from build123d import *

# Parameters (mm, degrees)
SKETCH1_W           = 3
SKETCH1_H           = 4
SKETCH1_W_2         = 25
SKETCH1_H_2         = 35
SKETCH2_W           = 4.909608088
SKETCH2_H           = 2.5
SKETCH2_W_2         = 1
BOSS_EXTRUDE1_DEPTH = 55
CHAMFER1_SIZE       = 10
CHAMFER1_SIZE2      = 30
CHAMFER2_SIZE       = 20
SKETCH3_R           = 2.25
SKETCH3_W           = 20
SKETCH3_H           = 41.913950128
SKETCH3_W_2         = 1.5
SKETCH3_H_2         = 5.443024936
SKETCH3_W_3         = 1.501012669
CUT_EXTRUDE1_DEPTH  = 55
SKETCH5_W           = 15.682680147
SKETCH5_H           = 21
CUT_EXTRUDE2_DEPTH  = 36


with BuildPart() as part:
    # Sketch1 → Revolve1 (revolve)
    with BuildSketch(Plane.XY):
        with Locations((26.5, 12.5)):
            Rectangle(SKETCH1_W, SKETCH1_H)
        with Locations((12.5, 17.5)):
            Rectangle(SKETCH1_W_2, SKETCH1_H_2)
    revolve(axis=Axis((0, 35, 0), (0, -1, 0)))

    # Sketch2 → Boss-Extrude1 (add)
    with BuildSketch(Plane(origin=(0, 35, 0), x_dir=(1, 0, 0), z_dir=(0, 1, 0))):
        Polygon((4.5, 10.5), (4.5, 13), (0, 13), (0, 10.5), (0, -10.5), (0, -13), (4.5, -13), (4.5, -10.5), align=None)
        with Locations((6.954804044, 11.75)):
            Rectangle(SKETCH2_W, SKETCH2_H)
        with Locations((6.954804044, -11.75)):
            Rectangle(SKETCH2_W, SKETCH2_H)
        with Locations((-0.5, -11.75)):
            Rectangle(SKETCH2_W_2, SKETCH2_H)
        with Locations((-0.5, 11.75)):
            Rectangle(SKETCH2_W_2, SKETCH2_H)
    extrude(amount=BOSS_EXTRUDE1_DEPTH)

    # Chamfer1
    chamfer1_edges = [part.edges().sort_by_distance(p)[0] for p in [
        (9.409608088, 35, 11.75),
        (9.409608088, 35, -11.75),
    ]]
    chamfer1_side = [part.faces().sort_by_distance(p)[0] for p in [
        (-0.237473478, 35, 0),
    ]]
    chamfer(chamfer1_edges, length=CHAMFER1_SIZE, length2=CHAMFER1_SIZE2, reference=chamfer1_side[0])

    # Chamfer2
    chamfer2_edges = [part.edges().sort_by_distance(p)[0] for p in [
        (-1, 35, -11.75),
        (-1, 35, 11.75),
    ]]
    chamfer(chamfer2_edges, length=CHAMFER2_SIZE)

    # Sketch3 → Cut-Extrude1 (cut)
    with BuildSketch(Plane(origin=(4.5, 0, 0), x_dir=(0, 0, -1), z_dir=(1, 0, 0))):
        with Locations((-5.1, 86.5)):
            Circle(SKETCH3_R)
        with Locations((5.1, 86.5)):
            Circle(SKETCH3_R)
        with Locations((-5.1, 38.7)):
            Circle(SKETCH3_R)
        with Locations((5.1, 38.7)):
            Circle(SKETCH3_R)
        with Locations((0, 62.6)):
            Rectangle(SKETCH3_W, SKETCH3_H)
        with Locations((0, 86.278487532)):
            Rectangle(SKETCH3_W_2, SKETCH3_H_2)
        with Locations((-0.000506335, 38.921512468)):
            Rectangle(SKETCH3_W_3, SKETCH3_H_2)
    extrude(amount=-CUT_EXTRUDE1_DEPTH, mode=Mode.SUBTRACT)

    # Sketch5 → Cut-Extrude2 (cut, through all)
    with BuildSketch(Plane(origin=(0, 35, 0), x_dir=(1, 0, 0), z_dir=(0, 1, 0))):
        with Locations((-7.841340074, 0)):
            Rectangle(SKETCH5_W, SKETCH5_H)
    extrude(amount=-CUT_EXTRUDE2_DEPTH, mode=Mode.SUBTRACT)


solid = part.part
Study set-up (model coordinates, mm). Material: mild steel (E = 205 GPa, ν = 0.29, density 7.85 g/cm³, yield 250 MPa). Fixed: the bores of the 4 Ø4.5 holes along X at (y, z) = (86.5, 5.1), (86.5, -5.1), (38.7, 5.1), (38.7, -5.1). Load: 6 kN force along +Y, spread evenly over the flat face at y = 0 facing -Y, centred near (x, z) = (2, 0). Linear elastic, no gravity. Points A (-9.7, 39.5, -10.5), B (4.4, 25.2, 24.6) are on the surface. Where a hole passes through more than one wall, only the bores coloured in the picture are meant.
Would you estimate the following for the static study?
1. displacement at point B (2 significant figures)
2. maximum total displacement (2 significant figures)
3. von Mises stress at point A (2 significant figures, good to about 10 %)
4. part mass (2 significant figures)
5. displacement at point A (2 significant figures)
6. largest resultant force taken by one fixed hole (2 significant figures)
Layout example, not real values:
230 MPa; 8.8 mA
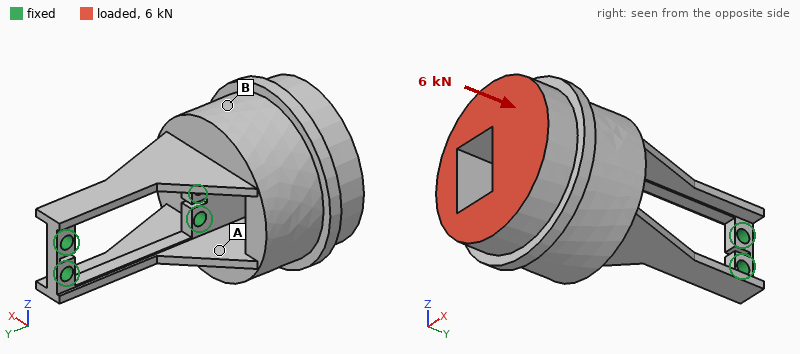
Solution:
2.8 µm; 10.0 µm; 13 MPa; 510 g; 4.8 µm; 2.9 kN
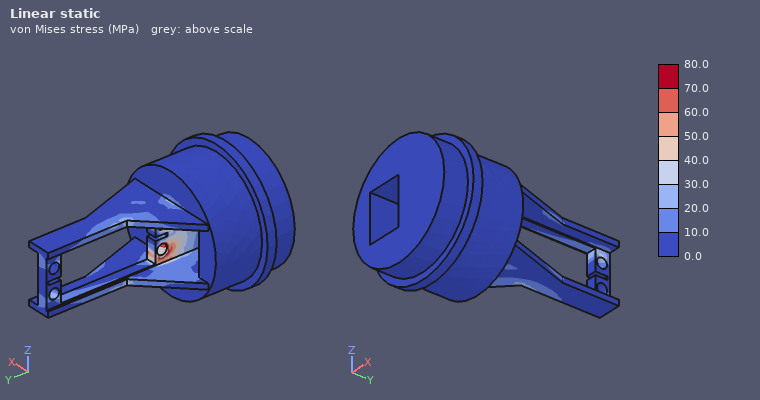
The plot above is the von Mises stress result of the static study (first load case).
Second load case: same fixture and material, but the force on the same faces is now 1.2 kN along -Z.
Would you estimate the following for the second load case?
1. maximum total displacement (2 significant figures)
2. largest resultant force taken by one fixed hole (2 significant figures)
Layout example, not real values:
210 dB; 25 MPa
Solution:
19 µm; 2.6 kN
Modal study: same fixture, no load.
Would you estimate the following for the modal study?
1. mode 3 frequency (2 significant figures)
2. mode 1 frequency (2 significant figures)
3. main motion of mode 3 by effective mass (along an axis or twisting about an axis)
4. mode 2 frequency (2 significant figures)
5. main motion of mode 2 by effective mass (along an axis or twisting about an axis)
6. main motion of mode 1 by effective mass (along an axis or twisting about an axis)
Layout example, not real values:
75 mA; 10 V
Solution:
3200 Hz; 1700 Hz; along Z; 2700 Hz; along Z; along X
